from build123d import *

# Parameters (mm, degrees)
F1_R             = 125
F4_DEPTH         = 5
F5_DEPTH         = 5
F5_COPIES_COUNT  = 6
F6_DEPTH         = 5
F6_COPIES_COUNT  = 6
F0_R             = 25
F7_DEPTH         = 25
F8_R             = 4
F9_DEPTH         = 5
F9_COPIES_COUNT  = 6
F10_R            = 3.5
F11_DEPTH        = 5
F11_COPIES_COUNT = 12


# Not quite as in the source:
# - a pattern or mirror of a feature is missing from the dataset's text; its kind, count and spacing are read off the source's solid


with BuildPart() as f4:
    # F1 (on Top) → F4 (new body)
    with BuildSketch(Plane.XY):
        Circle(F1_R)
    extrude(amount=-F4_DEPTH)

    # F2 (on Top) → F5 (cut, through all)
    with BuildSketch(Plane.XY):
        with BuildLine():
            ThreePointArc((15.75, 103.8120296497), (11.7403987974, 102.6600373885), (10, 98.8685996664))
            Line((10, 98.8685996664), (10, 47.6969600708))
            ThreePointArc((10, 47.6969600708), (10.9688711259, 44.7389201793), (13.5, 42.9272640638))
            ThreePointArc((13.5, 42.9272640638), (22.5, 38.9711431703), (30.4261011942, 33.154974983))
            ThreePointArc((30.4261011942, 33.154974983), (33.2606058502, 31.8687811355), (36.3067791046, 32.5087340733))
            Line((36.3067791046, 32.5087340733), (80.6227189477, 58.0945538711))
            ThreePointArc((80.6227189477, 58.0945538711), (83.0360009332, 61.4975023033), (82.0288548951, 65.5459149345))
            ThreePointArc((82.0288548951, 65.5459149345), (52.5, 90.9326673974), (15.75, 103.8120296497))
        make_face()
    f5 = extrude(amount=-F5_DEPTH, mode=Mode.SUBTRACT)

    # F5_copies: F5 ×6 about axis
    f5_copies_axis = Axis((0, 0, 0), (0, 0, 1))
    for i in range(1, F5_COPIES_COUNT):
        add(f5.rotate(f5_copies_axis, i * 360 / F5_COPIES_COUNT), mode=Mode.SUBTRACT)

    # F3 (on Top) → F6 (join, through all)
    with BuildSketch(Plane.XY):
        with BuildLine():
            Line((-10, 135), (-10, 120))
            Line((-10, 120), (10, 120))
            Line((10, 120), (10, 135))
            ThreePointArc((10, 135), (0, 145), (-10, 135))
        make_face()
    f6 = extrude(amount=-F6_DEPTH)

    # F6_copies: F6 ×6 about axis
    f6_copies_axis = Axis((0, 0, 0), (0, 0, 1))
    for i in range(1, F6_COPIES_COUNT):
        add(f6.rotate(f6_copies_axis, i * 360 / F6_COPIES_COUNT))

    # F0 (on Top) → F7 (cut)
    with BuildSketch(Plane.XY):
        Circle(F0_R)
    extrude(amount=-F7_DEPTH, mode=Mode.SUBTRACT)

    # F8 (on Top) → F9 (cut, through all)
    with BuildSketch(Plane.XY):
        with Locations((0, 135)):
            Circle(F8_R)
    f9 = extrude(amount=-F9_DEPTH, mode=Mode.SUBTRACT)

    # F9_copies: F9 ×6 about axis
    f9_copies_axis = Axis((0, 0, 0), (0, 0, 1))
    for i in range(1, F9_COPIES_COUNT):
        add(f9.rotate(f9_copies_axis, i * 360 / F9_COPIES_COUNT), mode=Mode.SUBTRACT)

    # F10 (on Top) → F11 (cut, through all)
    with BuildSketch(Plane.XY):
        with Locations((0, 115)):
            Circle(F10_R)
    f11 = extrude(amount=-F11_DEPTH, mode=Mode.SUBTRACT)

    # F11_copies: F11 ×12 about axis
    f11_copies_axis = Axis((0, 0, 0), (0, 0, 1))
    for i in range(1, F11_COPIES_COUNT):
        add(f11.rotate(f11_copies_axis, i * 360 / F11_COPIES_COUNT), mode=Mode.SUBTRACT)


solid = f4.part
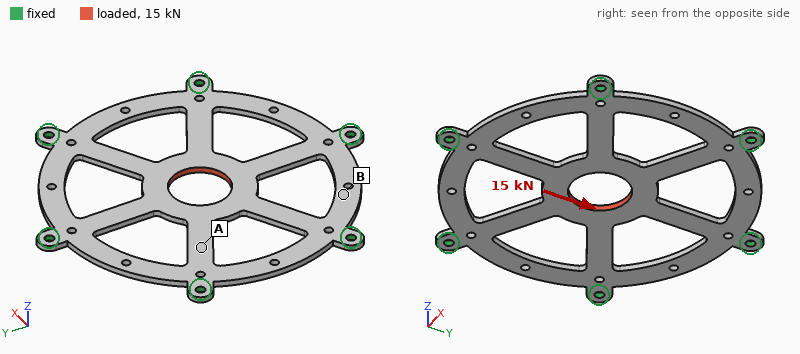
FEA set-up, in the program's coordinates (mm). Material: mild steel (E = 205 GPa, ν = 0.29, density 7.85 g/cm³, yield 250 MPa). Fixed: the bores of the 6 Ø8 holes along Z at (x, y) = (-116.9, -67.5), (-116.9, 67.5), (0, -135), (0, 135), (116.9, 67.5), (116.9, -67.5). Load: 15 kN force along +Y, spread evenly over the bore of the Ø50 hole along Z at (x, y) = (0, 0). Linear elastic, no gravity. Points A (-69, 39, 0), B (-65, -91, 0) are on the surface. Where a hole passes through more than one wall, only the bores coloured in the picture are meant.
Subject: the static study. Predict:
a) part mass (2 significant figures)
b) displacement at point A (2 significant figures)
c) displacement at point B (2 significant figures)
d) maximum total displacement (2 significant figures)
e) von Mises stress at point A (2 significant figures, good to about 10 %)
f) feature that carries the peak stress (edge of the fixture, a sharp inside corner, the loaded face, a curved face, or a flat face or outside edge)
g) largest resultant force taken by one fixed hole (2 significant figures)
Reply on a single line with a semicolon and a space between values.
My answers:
1.1 kg; 12 µm; 6.0 µm; 25 µm; 24 MPa; a curved face; 4.6 kN
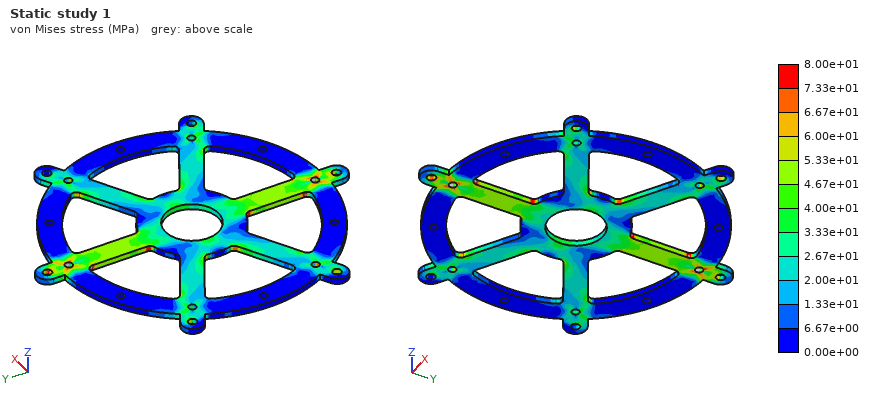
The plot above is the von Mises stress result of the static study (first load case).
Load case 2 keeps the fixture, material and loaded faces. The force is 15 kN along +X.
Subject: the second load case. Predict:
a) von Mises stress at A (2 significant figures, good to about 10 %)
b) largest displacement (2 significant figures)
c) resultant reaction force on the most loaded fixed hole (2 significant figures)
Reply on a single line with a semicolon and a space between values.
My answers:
41 MPa; 26 µm; 4.0 kN
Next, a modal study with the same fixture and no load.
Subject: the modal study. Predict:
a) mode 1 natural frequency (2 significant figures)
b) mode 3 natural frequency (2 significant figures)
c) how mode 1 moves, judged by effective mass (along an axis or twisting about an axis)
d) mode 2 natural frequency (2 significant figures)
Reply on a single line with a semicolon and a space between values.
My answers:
470 Hz; 1100 Hz; along Z; 1100 Hz
